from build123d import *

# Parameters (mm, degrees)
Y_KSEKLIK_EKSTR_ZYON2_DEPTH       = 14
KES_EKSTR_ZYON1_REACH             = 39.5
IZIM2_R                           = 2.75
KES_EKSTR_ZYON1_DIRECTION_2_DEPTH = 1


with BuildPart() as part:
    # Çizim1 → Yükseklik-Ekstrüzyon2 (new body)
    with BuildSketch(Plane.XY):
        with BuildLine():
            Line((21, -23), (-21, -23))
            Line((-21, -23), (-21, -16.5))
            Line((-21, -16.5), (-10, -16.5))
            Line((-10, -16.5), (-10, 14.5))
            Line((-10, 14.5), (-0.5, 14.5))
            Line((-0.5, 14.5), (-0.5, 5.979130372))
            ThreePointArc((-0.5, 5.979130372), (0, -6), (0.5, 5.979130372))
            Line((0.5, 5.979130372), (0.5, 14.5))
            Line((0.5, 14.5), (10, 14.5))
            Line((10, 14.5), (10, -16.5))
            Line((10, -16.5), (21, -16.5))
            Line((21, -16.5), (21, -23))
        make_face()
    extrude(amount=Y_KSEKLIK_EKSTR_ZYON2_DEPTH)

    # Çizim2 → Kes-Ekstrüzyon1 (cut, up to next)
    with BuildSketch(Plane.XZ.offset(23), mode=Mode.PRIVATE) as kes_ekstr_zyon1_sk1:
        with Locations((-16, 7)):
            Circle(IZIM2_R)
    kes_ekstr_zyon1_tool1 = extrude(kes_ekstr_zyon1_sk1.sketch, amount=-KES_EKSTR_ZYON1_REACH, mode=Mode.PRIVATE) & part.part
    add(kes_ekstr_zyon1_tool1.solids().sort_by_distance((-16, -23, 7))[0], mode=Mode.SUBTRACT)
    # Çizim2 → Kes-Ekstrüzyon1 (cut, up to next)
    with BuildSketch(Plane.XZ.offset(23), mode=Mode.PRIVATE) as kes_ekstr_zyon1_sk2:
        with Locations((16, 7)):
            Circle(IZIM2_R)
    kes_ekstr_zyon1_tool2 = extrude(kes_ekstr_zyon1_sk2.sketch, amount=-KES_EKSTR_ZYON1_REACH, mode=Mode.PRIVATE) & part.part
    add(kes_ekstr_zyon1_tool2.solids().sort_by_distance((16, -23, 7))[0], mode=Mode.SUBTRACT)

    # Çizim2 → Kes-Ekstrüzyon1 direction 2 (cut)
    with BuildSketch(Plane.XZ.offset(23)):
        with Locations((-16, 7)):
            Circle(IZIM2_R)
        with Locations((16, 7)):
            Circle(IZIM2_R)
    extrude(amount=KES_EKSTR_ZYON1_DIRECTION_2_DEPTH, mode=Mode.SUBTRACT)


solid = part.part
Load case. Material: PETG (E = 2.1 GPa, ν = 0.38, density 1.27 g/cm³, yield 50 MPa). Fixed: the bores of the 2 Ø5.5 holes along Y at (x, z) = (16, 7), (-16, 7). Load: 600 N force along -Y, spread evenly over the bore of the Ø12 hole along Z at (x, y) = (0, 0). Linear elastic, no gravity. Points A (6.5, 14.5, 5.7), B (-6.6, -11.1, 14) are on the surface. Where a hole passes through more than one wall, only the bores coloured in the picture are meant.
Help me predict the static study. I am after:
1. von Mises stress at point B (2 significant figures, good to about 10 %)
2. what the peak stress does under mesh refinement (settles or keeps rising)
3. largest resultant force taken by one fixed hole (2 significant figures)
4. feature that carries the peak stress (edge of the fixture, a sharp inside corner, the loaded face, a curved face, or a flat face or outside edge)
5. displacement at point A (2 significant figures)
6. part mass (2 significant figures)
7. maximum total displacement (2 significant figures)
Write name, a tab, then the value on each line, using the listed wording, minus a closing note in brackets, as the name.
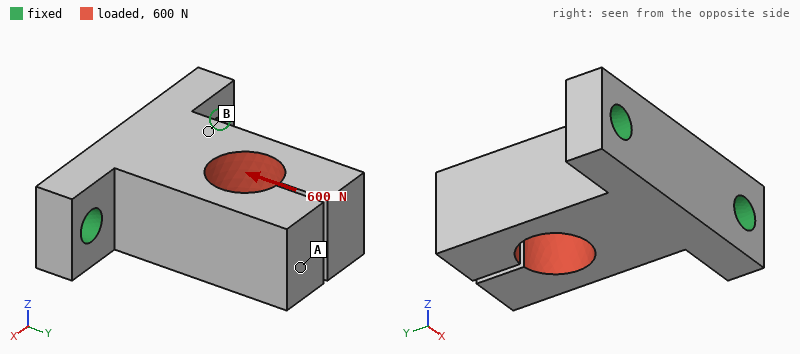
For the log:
von Mises stress at point B	4.1 MPa
what the peak stress does under mesh refinement	keeps rising
largest resultant force taken by one fixed hole	320 N
feature that carries the peak stress	edge of the fixture
displacement at point A	0.45 mm
part mass	13 g
maximum total displacement	0.52 mm
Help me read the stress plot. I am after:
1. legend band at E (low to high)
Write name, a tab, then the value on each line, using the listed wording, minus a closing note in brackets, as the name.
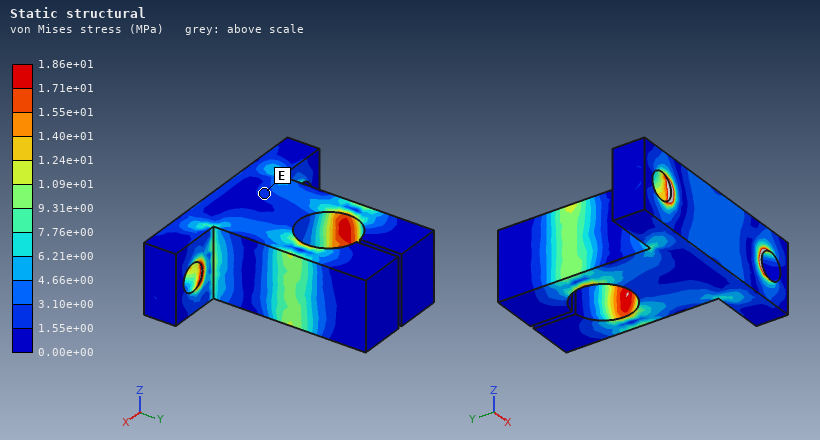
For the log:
legend band at E	1.55e+00 to 3.10e+00 MPa
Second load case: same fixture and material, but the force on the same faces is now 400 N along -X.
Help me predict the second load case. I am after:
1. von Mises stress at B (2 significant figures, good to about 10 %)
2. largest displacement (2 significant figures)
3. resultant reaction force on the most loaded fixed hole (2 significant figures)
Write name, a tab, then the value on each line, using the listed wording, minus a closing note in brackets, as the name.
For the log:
von Mises stress at B	2.0 MPa
largest displacement	0.68 mm
resultant reaction force on the most loaded fixed hole	370 N
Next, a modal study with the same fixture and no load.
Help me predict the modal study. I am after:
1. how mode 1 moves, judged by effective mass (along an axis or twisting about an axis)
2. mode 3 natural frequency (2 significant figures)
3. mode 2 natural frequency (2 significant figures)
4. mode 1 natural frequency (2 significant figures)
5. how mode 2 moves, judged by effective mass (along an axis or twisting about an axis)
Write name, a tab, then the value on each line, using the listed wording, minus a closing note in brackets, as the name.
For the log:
how mode 1 moves, judged by effective mass	along Z
mode 3 natural frequency	1400 Hz
mode 2 natural frequency	1300 Hz
mode 1 natural frequency	1100 Hz
how mode 2 moves, judged by effective mass	along X
